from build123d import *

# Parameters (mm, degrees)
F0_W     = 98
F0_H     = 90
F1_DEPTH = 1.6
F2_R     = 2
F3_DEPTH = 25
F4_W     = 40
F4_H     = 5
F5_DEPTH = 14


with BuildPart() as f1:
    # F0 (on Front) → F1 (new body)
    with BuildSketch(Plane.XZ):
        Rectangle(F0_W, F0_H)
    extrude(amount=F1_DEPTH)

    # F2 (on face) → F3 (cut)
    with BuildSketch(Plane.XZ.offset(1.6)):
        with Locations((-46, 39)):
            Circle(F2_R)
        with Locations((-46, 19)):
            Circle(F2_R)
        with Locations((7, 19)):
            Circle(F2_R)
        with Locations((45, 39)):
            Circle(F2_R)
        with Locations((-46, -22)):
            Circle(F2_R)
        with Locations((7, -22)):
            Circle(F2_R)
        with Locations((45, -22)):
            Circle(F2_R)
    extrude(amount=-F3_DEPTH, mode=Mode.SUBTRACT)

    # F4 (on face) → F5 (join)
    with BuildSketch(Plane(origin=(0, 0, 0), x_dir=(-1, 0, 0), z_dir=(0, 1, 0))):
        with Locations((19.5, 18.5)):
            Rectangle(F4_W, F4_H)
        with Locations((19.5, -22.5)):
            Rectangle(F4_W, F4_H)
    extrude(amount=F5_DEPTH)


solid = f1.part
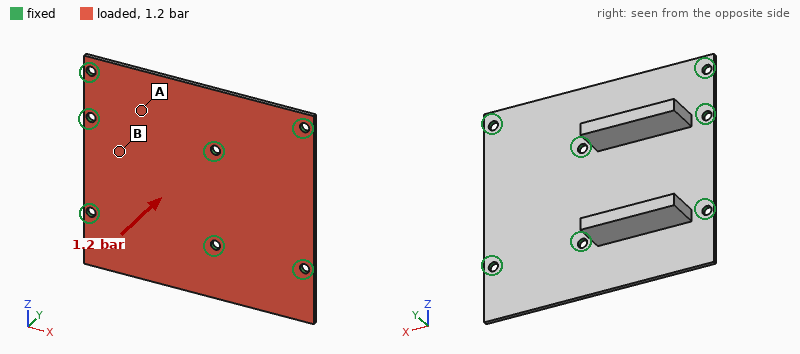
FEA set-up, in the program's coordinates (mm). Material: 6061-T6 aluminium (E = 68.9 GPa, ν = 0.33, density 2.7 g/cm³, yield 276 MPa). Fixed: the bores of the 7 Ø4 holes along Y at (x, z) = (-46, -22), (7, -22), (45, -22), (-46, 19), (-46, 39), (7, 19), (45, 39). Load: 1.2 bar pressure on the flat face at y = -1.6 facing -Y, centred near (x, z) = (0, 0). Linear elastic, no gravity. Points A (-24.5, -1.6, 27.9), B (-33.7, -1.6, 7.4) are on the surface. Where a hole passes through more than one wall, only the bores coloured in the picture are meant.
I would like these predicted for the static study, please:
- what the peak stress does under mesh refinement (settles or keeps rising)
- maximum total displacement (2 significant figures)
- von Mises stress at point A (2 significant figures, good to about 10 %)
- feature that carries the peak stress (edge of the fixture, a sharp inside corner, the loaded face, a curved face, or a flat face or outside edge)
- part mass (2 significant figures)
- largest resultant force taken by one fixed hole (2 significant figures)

keeps rising
0.19 mm
19 MPa
edge of the fixture
53 g
260 N
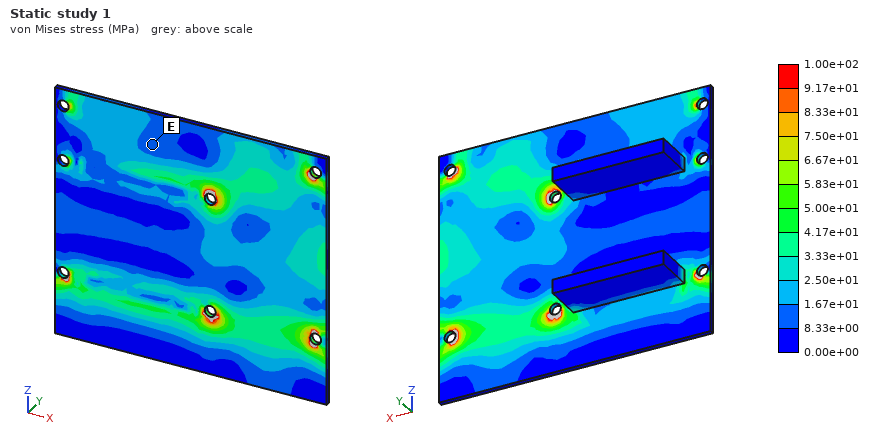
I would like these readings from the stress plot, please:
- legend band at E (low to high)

8.33e+00 to 1.67e+01 MPa
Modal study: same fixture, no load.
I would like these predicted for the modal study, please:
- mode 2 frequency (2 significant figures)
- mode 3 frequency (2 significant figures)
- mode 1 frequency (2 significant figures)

2400 Hz
2500 Hz
2100 Hz
